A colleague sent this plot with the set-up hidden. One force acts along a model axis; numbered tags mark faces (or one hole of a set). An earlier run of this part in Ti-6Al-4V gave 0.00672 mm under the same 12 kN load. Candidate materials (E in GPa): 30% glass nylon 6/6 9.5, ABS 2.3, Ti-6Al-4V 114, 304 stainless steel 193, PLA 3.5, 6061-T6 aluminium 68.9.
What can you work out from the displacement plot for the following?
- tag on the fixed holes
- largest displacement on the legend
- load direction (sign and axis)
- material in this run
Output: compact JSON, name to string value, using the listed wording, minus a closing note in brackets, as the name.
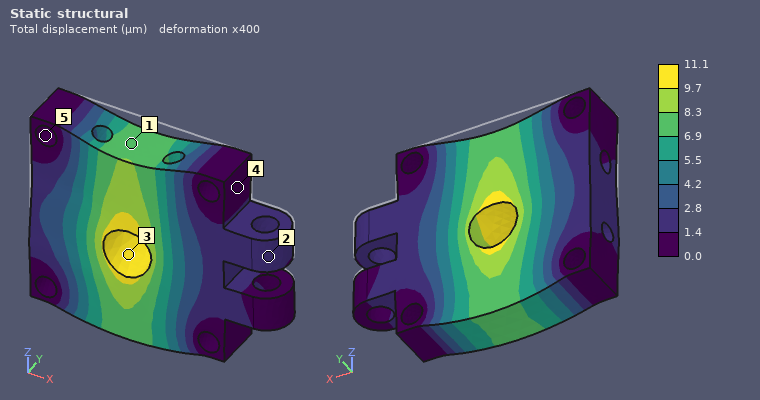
{"tag on the fixed holes": "5", "largest displacement on the legend": "11.1 µm", "load direction": "-Z", "material in this run": "6061-T6 aluminium"}
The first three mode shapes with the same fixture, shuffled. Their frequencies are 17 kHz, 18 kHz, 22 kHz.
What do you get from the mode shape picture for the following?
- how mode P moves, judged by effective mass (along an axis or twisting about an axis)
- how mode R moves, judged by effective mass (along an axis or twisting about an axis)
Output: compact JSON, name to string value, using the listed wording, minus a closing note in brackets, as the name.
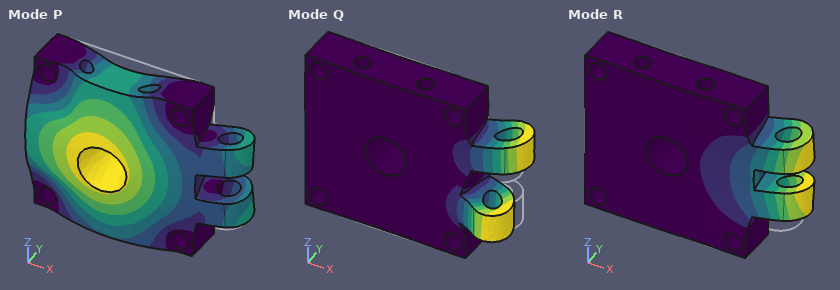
{"how mode P moves, judged by effective mass": "along Y", "how mode R moves, judged by effective mass": "along Y"}
